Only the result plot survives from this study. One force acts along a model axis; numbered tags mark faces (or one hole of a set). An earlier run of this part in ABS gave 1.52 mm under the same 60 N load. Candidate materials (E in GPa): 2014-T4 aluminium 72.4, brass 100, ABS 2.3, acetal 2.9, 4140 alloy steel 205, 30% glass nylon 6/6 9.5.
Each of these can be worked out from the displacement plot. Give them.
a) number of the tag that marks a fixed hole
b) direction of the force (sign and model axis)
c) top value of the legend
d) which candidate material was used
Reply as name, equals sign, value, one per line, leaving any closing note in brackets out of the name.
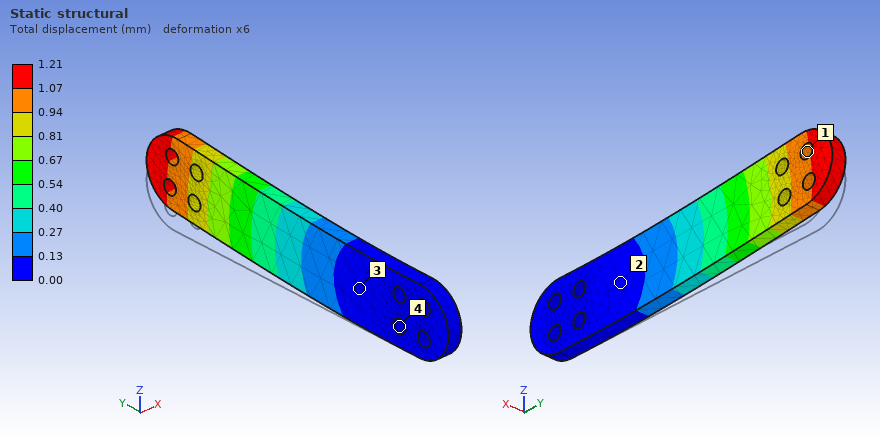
number of the tag that marks a fixed hole = 4
direction of the force = +Z
top value of the legend = 1.21 mm
which candidate material was used = acetal
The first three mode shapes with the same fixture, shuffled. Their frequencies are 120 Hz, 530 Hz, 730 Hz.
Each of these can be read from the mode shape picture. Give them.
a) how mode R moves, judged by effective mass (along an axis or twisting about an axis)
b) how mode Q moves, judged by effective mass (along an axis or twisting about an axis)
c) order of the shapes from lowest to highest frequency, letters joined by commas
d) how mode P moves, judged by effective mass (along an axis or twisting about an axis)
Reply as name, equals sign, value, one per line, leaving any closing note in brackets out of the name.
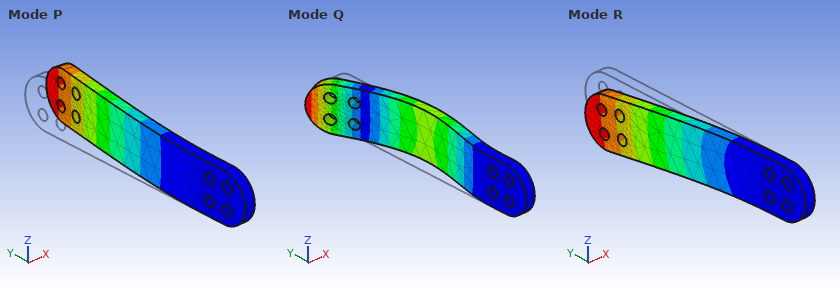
how mode R moves, judged by effective mass = along Z
how mode Q moves, judged by effective mass = along X
order of the shapes from lowest to highest frequency, letters joined by commas = P, R, Q
how mode P moves, judged by effective mass = along X
